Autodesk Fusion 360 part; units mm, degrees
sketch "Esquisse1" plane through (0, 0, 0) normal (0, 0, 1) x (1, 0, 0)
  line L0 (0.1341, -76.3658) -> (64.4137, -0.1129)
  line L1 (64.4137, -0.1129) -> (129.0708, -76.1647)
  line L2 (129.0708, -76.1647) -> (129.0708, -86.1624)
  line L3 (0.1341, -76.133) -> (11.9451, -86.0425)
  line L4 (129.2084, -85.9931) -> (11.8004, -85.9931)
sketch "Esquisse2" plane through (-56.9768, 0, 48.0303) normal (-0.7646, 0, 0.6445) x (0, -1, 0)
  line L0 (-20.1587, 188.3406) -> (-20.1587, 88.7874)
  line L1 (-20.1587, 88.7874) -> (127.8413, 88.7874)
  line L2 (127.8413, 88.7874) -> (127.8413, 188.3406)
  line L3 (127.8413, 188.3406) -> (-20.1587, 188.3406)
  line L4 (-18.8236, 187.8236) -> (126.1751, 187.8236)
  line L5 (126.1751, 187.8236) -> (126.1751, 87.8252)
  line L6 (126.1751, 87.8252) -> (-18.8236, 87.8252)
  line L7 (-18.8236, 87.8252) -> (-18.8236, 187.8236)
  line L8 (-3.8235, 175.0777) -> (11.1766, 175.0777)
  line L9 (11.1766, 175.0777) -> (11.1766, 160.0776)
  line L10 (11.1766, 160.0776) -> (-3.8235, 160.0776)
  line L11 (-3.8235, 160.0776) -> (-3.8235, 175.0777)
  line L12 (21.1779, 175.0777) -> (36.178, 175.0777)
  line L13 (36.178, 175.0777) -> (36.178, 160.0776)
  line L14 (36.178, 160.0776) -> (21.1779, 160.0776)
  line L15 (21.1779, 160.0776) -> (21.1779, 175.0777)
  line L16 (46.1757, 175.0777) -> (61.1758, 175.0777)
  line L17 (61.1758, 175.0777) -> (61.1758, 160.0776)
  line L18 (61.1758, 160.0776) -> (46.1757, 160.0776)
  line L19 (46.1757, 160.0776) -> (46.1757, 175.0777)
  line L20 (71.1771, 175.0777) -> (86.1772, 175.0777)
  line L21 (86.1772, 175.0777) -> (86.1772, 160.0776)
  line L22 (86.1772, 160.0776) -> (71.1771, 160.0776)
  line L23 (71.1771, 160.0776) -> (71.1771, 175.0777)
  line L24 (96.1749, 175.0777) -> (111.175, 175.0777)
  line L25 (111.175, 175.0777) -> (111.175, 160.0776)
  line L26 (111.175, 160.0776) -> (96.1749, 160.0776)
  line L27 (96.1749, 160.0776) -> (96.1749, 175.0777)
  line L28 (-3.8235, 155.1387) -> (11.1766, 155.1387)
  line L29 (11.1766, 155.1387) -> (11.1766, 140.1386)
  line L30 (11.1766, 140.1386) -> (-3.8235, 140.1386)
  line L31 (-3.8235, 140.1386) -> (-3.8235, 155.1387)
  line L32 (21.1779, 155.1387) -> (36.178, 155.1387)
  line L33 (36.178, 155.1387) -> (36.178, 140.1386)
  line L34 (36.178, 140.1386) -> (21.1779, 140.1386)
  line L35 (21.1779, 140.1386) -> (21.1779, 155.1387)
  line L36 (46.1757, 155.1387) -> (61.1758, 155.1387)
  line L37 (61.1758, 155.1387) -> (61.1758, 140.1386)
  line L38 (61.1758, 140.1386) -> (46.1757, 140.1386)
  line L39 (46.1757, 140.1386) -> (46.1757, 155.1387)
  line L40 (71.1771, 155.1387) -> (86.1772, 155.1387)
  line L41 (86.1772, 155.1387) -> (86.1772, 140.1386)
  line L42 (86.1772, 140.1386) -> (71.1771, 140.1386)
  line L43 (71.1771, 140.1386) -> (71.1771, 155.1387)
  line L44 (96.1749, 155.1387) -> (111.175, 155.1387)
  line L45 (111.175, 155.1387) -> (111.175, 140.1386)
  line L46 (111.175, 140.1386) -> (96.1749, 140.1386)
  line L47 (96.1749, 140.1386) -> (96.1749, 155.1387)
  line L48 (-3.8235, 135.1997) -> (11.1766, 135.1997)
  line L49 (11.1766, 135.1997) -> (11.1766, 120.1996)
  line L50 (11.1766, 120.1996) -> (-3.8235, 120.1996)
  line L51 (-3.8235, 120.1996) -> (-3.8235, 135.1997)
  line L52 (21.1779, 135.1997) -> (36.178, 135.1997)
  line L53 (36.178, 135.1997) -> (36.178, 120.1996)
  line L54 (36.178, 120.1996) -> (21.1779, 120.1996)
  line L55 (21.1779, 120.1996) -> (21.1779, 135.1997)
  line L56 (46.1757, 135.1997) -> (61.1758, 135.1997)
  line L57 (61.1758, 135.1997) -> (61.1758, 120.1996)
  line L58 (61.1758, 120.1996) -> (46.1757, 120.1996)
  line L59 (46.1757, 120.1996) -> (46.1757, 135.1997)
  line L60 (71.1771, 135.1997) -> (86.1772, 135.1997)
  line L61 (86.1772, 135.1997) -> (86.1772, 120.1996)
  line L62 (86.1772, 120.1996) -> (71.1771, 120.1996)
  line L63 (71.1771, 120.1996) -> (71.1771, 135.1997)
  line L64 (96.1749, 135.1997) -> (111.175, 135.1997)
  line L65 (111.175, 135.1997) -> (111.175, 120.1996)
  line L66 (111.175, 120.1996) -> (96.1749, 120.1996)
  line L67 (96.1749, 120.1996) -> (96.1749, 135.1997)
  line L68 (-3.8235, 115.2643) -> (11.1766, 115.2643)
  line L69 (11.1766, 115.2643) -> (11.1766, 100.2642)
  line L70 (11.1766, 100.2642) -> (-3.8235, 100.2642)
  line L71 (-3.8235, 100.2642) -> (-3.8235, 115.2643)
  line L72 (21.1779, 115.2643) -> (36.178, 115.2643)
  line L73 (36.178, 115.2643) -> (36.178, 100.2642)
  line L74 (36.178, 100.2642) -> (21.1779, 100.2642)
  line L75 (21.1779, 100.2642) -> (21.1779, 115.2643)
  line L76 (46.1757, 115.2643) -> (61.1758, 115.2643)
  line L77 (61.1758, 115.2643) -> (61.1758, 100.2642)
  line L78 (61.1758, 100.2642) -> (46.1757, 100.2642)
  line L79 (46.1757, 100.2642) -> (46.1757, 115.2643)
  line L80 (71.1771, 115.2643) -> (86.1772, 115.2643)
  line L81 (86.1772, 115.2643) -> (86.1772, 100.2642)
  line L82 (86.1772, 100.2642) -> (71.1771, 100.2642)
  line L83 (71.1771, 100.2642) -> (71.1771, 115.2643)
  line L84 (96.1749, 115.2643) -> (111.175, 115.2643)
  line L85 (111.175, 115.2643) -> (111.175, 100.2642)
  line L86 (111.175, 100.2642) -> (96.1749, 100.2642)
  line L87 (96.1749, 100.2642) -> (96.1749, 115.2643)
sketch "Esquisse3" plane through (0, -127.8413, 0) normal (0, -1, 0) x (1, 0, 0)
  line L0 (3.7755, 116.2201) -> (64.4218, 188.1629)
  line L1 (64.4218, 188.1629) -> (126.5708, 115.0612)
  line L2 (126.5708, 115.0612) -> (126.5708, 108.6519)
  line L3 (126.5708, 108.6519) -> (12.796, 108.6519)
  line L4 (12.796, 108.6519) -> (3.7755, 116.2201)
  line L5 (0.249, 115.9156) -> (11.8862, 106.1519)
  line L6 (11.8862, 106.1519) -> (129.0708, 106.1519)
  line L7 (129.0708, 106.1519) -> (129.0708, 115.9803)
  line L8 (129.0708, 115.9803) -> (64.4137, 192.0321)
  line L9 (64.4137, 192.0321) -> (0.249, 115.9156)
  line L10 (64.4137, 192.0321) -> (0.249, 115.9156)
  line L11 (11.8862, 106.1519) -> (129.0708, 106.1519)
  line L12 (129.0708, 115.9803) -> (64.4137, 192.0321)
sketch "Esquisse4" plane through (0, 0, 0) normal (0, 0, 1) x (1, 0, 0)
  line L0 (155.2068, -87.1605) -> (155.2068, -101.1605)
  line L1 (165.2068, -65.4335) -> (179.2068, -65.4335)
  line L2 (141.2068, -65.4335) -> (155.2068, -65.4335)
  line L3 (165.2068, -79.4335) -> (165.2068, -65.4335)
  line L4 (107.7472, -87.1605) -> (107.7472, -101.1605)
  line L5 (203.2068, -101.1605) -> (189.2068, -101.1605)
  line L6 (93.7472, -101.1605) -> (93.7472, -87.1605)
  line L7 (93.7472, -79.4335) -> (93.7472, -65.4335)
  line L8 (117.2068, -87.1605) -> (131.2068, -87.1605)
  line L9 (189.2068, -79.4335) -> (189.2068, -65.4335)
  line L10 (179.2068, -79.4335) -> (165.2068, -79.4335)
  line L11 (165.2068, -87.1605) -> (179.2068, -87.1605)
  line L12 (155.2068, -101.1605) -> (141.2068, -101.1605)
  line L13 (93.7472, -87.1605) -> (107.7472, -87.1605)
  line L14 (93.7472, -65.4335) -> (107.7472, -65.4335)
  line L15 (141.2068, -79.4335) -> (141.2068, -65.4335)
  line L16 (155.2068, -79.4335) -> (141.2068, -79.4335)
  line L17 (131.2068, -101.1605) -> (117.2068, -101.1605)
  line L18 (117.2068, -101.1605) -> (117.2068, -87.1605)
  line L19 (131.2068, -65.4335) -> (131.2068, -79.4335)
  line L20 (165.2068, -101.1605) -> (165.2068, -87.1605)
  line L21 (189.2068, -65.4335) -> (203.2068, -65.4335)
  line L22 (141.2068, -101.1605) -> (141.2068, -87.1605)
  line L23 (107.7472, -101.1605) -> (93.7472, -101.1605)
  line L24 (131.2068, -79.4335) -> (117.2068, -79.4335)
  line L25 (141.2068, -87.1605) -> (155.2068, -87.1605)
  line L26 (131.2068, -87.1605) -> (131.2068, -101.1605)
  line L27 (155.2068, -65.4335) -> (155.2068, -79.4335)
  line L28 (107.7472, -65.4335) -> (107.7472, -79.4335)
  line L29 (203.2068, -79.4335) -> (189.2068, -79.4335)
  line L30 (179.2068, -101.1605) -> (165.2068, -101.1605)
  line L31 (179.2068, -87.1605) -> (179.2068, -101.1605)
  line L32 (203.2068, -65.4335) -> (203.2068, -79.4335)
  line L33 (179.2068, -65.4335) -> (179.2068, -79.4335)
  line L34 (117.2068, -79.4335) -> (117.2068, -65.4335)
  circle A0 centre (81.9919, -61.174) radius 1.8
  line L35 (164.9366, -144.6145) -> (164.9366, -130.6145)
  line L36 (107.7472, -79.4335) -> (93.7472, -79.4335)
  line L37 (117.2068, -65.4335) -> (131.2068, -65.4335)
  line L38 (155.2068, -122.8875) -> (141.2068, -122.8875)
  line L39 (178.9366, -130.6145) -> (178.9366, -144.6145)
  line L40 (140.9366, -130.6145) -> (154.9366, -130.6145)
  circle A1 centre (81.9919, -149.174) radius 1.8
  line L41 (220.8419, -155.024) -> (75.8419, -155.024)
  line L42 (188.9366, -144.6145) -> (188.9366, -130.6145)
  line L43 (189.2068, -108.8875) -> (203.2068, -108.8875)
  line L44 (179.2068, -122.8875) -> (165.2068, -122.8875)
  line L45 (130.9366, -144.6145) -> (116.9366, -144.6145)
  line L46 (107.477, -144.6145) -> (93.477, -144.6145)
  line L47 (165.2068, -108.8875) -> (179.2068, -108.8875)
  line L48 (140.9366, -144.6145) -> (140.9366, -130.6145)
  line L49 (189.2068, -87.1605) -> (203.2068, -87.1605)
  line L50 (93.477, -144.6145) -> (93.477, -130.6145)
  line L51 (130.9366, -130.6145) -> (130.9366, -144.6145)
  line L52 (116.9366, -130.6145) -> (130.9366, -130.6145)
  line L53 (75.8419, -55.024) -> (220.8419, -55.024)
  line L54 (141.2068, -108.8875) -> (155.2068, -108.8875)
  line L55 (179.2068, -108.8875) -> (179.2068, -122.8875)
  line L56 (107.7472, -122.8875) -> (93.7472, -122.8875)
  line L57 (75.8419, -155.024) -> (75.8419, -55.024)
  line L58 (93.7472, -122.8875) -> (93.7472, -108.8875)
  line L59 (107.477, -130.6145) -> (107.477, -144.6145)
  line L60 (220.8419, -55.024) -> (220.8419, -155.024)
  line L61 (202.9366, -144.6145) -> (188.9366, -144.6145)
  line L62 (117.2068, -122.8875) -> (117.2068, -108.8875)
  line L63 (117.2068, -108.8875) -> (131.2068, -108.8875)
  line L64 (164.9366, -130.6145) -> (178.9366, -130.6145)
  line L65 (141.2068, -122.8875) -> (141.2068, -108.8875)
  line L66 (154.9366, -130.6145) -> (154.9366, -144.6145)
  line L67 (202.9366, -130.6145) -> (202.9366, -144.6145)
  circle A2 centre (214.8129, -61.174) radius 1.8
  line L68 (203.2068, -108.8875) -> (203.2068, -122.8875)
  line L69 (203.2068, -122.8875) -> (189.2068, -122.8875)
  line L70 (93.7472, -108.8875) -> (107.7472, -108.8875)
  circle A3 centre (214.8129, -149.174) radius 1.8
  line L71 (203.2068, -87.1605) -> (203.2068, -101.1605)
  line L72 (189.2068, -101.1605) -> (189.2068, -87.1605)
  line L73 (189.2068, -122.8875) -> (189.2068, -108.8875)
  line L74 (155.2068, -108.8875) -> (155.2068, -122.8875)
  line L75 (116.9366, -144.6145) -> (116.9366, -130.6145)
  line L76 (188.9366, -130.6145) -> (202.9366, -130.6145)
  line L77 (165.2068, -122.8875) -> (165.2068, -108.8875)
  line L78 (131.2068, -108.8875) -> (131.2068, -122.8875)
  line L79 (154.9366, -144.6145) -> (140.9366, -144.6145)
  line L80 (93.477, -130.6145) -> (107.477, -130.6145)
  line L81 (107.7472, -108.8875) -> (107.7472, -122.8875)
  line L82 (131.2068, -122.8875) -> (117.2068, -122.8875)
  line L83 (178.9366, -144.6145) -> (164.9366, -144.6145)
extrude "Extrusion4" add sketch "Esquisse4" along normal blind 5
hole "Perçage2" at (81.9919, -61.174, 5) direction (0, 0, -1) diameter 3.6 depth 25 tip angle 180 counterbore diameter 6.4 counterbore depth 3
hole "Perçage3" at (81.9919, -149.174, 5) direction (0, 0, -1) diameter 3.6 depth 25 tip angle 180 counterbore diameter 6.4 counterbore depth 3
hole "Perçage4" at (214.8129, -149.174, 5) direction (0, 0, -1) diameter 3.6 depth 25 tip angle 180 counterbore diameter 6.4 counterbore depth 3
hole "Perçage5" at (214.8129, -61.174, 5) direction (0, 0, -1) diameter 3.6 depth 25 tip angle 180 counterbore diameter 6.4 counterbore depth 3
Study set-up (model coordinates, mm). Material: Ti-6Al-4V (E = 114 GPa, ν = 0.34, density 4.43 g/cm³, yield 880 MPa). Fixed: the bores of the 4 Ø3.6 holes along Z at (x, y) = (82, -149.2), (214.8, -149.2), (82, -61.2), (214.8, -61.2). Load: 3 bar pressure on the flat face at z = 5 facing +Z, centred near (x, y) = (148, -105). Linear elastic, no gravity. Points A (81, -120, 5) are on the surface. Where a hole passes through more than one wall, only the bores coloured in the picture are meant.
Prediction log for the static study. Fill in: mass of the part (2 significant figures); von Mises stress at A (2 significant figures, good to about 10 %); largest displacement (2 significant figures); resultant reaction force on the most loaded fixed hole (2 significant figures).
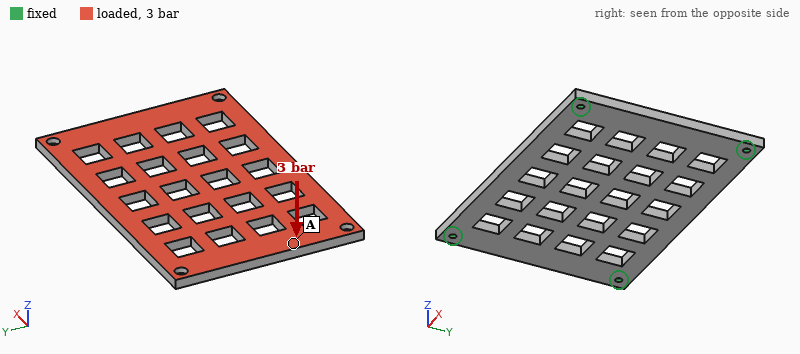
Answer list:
230 g
45 MPa
0.57 mm
1.8 kN
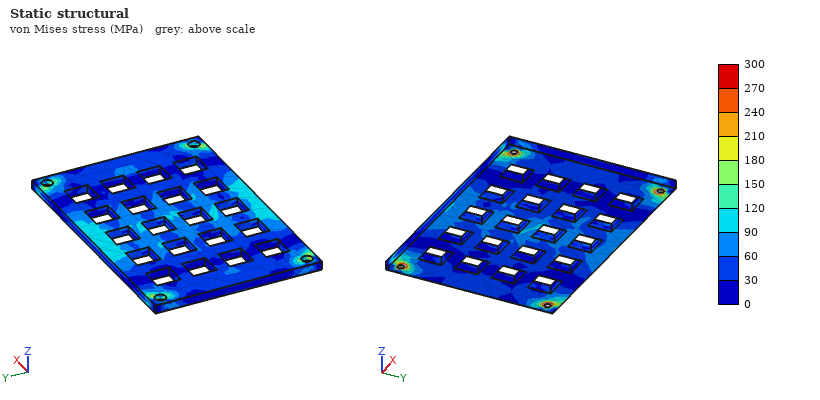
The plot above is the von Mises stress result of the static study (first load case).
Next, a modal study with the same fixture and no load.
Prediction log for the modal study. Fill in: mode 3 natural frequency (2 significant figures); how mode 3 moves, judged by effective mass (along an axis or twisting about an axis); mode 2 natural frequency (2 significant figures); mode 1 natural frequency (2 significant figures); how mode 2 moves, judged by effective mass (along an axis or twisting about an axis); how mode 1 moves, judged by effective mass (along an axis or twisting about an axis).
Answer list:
2200 Hz
twisting about Y
1500 Hz
910 Hz
twisting about X
along Z
